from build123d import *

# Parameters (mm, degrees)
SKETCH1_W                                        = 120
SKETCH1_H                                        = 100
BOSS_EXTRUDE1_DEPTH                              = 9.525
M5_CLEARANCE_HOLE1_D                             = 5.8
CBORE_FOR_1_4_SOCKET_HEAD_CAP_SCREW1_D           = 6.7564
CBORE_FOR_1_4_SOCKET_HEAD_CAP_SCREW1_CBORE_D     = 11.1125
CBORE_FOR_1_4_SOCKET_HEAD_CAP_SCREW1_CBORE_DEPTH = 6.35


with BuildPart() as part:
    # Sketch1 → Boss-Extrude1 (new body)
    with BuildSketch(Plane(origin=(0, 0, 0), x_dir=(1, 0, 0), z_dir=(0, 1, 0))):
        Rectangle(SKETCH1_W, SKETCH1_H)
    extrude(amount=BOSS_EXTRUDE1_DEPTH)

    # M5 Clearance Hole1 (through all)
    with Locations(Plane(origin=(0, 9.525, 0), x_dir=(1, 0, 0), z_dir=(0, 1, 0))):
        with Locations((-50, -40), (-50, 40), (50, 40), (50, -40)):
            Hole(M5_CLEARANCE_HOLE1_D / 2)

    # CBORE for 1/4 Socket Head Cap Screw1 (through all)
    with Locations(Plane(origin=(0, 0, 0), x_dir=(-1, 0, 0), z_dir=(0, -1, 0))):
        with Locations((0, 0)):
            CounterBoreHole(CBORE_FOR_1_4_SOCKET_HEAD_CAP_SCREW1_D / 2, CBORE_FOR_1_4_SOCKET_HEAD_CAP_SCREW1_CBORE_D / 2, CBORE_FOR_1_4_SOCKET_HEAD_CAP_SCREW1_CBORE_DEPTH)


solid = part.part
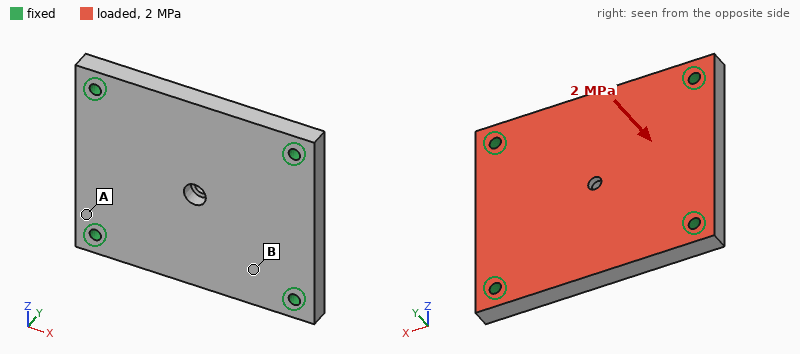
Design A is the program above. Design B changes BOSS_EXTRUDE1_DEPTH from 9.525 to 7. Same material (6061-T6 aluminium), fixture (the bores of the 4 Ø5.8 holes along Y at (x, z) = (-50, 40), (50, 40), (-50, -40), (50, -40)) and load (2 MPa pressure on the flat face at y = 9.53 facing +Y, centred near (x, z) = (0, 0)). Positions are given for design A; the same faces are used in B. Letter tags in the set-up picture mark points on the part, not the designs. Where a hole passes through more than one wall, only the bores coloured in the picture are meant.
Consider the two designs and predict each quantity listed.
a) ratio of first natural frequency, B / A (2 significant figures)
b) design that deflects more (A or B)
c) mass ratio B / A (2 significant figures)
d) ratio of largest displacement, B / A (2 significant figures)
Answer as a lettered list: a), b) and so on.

a) 0.77
b) B
c) 0.73
d) 2.3
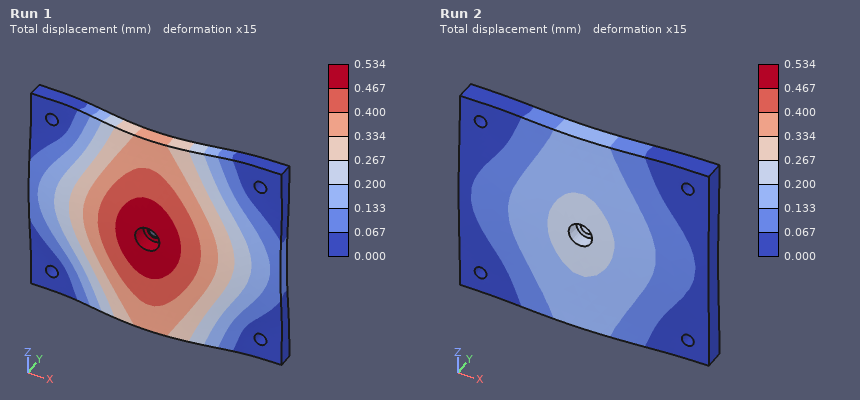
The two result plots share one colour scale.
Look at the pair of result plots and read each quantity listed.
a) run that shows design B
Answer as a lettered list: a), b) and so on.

a) Run 1
